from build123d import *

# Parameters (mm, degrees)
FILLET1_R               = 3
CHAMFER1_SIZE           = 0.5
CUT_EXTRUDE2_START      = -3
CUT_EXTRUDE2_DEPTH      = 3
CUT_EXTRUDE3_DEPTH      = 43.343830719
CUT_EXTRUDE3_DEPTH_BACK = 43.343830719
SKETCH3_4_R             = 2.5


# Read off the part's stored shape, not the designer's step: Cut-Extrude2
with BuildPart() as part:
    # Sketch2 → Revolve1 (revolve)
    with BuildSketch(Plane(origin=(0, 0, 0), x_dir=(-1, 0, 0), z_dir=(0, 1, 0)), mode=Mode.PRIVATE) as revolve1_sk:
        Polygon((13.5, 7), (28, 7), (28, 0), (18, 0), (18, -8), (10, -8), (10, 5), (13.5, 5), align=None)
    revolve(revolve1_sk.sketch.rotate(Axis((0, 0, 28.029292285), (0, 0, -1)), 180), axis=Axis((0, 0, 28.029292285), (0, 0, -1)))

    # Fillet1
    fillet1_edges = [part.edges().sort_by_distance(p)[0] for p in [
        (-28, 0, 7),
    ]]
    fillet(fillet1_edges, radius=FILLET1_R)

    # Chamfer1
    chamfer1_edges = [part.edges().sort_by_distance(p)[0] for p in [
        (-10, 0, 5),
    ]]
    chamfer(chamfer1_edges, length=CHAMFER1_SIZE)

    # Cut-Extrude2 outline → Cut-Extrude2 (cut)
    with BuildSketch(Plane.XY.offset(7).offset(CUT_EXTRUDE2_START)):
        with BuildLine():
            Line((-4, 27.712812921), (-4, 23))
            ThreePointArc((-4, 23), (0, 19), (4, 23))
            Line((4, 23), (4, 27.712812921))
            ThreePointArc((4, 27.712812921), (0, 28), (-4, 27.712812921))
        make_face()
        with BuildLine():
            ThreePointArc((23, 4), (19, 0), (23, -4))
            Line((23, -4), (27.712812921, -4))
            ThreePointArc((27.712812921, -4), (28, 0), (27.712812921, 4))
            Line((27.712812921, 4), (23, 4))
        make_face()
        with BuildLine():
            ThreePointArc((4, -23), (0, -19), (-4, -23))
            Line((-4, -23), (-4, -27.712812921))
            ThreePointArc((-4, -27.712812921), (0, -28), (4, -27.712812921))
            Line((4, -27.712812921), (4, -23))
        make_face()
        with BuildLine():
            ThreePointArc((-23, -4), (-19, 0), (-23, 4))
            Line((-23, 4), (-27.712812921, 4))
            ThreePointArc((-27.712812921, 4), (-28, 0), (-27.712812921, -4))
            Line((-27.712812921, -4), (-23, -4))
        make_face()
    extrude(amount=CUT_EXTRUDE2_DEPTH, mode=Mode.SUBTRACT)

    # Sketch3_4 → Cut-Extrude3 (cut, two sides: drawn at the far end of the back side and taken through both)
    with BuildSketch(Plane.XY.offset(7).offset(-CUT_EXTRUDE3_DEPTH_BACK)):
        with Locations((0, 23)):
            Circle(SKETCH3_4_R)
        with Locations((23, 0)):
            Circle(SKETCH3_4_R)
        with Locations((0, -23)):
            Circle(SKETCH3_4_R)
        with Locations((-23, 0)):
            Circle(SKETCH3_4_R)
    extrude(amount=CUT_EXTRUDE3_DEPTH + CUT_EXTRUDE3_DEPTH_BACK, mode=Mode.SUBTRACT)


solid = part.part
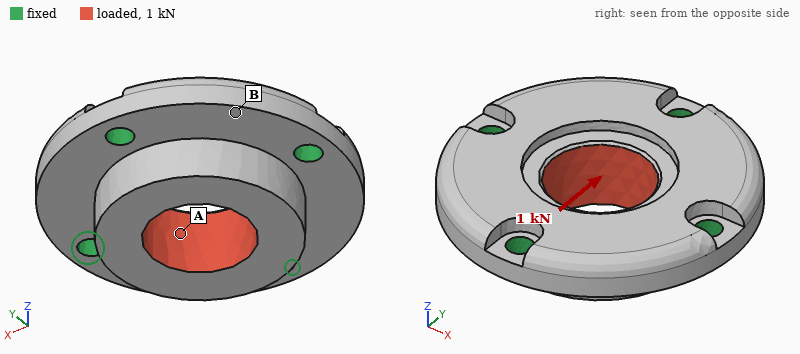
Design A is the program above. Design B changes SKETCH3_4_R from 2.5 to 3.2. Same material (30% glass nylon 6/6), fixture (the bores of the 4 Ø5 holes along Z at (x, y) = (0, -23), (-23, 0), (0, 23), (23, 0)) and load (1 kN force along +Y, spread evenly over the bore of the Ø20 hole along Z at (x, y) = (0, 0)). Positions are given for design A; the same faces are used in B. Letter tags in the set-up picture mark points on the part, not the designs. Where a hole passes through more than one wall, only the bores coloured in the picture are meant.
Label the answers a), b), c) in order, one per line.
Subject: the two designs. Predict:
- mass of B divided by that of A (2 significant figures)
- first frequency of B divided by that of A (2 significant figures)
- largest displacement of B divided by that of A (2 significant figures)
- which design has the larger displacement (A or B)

a) 0.99
b) 1.1
c) 0.90
d) A
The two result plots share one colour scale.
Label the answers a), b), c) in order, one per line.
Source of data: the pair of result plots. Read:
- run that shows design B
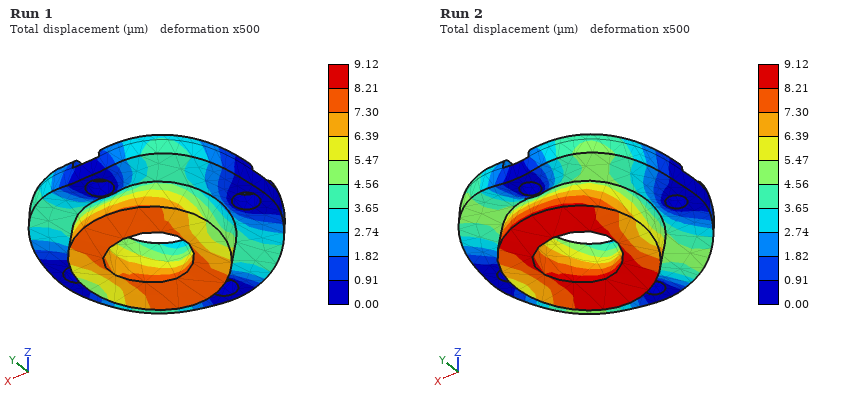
a) Run 1
